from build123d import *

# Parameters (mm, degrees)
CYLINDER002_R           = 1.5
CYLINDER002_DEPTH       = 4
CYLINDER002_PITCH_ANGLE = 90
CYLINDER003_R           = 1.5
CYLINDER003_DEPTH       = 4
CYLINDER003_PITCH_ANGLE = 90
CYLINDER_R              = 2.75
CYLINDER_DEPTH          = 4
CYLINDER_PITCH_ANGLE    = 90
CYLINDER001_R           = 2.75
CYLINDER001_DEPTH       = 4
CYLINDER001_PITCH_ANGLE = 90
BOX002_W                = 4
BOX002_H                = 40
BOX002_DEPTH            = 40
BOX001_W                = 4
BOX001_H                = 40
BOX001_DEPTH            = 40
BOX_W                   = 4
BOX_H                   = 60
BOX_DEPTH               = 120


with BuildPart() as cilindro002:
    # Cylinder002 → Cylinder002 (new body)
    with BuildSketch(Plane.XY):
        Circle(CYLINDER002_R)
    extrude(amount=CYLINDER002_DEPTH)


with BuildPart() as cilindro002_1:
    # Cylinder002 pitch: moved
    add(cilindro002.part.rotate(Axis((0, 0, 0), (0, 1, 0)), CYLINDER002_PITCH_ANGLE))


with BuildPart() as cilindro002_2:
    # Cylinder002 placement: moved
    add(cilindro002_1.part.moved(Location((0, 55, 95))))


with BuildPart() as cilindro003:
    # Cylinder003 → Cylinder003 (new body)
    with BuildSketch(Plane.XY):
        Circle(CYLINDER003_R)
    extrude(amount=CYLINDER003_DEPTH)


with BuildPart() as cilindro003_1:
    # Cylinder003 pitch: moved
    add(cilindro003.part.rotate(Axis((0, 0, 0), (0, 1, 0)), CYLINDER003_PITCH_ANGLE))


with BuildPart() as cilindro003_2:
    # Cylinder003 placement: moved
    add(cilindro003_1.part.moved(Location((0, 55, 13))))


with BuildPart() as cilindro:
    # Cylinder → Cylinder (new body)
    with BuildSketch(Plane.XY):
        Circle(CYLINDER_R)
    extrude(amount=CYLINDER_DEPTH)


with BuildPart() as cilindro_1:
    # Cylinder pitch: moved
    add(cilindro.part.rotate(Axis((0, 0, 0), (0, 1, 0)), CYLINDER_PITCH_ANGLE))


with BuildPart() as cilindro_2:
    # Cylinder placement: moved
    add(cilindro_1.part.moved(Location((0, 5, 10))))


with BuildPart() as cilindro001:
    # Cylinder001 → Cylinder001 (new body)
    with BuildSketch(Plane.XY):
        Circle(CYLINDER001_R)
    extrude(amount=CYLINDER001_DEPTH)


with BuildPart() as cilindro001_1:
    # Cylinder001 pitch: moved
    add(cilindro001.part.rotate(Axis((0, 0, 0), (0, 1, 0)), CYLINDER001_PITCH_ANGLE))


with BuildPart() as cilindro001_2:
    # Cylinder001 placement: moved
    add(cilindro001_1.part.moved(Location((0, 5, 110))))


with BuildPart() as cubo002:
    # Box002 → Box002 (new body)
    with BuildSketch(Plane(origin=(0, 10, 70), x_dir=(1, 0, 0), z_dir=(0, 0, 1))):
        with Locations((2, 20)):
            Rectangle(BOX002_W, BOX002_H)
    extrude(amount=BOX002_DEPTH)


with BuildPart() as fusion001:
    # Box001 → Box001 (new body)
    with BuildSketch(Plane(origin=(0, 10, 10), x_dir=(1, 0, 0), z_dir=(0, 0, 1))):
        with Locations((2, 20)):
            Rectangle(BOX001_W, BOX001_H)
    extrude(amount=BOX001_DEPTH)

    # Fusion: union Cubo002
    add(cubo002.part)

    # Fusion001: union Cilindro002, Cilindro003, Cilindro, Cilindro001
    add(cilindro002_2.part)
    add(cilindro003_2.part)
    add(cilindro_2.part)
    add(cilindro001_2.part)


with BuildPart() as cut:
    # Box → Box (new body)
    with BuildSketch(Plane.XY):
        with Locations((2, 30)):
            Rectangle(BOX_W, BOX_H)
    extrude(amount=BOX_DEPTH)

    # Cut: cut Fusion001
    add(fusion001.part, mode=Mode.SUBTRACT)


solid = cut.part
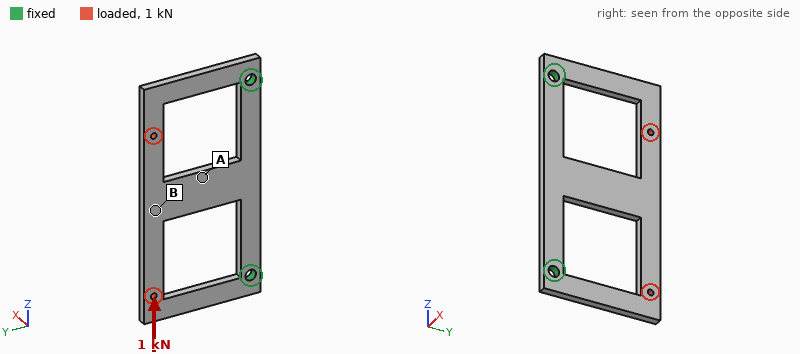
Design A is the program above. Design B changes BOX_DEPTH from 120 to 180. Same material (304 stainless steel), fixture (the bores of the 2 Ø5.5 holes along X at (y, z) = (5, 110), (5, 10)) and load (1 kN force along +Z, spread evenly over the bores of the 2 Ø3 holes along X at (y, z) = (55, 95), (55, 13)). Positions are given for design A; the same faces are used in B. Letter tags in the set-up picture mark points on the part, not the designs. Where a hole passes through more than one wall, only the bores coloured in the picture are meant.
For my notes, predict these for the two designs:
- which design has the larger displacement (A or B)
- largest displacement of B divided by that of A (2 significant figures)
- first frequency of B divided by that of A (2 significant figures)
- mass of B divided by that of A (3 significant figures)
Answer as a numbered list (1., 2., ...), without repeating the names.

1. B
2. 1.4
3. 0.66
4. 1.91
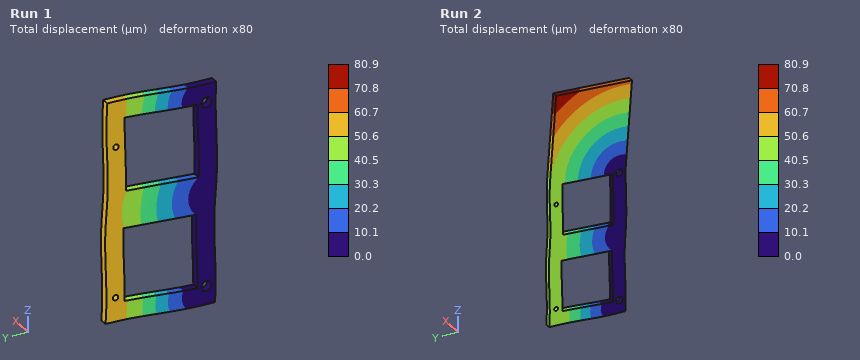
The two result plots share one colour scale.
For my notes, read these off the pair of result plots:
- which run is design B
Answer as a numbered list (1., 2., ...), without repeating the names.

1. Run 2
